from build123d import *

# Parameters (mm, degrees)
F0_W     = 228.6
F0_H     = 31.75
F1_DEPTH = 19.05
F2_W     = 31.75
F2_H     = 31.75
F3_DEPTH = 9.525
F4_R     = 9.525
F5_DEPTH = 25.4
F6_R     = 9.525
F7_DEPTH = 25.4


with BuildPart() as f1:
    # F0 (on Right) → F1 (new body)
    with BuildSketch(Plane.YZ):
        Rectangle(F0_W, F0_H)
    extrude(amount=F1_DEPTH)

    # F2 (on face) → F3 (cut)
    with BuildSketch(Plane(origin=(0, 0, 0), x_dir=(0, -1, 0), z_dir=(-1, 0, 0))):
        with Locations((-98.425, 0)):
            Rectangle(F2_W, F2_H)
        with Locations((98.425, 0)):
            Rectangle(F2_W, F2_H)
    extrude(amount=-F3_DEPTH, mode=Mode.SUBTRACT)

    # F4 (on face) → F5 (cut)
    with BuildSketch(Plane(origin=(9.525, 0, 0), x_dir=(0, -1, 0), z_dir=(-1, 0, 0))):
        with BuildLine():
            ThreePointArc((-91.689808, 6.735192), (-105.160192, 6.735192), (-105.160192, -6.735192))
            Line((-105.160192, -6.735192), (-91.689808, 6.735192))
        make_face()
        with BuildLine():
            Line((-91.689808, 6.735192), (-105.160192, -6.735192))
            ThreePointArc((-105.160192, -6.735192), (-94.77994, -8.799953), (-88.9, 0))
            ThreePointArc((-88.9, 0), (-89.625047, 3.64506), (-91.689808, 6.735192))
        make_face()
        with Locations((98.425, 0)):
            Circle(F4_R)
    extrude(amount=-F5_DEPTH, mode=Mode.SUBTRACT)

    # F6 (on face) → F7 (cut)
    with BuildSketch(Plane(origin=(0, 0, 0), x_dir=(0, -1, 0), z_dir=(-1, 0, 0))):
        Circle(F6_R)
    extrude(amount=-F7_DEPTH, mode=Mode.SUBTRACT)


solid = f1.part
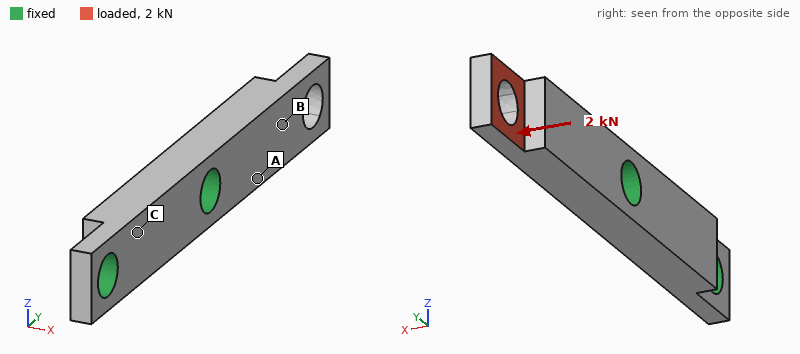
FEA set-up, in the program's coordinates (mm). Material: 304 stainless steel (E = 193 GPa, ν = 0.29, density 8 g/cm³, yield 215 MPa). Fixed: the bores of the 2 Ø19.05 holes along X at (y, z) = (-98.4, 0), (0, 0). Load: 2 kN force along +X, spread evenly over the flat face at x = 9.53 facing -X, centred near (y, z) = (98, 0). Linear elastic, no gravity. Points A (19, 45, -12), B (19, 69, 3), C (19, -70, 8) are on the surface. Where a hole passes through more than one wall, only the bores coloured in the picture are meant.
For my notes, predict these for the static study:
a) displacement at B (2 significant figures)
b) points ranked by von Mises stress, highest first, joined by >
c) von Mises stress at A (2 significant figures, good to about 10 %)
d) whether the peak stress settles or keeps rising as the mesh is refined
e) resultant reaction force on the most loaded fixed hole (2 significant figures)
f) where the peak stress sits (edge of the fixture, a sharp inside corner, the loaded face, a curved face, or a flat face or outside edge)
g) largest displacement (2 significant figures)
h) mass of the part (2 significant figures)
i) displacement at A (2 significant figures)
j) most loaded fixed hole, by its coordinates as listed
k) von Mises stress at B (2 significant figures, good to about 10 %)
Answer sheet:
0.084 mm
A > B > C
55 MPa
keeps rising
2.0 kN
edge of the fixture
0.23 mm
870 g
0.038 mm
(0, 0)
34 MPa
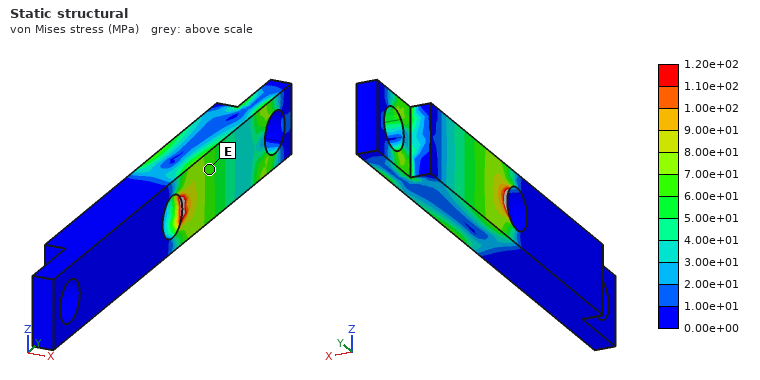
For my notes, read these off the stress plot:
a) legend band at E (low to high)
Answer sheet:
6.00e+01 to 7.00e+01 MPa
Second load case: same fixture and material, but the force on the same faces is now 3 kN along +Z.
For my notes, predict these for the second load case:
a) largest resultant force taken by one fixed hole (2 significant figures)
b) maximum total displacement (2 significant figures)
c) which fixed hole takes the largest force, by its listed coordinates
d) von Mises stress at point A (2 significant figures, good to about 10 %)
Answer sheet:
3.2 kN
0.15 mm
(0, 0)
38 MPa
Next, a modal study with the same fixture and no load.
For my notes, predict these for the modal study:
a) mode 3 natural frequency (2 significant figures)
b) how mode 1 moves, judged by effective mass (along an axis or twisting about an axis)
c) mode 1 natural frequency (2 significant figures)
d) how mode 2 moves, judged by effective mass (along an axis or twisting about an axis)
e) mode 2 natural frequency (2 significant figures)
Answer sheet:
5800 Hz
along X
1700 Hz
along Z
2500 Hz
